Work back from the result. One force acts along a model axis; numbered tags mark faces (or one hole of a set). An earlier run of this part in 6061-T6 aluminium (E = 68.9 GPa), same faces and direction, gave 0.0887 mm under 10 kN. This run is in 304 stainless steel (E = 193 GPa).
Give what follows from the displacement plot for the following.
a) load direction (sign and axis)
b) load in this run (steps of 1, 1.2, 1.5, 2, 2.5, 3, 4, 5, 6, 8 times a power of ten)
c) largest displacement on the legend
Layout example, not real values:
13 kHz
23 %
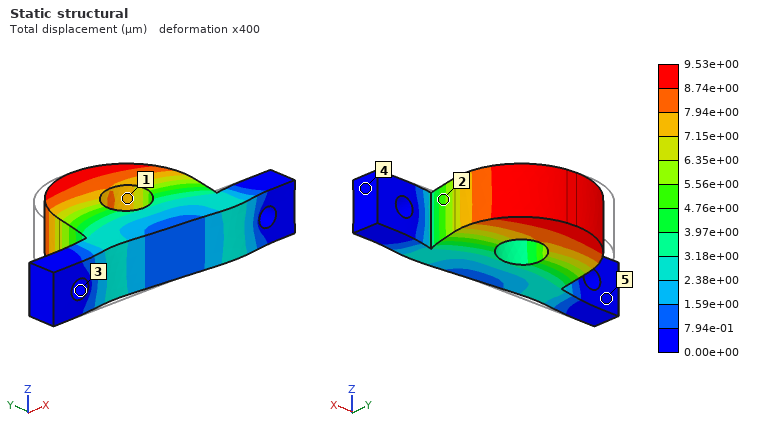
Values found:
+X
3 kN
9.53e+00 µm
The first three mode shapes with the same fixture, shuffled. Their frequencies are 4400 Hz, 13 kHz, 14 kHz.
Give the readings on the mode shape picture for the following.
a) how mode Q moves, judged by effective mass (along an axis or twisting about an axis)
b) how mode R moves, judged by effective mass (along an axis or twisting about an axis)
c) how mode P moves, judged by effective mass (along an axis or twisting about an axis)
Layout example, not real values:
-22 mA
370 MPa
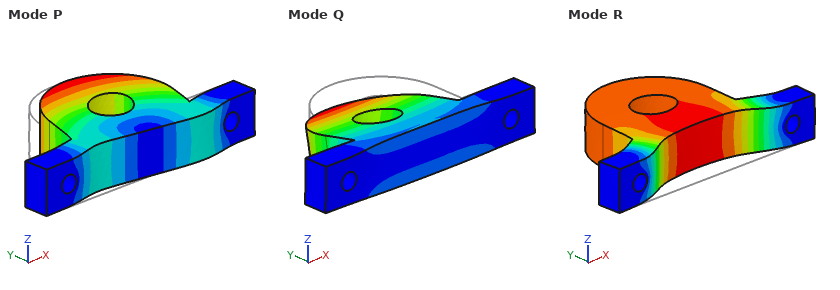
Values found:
along Z
along Y
along X
